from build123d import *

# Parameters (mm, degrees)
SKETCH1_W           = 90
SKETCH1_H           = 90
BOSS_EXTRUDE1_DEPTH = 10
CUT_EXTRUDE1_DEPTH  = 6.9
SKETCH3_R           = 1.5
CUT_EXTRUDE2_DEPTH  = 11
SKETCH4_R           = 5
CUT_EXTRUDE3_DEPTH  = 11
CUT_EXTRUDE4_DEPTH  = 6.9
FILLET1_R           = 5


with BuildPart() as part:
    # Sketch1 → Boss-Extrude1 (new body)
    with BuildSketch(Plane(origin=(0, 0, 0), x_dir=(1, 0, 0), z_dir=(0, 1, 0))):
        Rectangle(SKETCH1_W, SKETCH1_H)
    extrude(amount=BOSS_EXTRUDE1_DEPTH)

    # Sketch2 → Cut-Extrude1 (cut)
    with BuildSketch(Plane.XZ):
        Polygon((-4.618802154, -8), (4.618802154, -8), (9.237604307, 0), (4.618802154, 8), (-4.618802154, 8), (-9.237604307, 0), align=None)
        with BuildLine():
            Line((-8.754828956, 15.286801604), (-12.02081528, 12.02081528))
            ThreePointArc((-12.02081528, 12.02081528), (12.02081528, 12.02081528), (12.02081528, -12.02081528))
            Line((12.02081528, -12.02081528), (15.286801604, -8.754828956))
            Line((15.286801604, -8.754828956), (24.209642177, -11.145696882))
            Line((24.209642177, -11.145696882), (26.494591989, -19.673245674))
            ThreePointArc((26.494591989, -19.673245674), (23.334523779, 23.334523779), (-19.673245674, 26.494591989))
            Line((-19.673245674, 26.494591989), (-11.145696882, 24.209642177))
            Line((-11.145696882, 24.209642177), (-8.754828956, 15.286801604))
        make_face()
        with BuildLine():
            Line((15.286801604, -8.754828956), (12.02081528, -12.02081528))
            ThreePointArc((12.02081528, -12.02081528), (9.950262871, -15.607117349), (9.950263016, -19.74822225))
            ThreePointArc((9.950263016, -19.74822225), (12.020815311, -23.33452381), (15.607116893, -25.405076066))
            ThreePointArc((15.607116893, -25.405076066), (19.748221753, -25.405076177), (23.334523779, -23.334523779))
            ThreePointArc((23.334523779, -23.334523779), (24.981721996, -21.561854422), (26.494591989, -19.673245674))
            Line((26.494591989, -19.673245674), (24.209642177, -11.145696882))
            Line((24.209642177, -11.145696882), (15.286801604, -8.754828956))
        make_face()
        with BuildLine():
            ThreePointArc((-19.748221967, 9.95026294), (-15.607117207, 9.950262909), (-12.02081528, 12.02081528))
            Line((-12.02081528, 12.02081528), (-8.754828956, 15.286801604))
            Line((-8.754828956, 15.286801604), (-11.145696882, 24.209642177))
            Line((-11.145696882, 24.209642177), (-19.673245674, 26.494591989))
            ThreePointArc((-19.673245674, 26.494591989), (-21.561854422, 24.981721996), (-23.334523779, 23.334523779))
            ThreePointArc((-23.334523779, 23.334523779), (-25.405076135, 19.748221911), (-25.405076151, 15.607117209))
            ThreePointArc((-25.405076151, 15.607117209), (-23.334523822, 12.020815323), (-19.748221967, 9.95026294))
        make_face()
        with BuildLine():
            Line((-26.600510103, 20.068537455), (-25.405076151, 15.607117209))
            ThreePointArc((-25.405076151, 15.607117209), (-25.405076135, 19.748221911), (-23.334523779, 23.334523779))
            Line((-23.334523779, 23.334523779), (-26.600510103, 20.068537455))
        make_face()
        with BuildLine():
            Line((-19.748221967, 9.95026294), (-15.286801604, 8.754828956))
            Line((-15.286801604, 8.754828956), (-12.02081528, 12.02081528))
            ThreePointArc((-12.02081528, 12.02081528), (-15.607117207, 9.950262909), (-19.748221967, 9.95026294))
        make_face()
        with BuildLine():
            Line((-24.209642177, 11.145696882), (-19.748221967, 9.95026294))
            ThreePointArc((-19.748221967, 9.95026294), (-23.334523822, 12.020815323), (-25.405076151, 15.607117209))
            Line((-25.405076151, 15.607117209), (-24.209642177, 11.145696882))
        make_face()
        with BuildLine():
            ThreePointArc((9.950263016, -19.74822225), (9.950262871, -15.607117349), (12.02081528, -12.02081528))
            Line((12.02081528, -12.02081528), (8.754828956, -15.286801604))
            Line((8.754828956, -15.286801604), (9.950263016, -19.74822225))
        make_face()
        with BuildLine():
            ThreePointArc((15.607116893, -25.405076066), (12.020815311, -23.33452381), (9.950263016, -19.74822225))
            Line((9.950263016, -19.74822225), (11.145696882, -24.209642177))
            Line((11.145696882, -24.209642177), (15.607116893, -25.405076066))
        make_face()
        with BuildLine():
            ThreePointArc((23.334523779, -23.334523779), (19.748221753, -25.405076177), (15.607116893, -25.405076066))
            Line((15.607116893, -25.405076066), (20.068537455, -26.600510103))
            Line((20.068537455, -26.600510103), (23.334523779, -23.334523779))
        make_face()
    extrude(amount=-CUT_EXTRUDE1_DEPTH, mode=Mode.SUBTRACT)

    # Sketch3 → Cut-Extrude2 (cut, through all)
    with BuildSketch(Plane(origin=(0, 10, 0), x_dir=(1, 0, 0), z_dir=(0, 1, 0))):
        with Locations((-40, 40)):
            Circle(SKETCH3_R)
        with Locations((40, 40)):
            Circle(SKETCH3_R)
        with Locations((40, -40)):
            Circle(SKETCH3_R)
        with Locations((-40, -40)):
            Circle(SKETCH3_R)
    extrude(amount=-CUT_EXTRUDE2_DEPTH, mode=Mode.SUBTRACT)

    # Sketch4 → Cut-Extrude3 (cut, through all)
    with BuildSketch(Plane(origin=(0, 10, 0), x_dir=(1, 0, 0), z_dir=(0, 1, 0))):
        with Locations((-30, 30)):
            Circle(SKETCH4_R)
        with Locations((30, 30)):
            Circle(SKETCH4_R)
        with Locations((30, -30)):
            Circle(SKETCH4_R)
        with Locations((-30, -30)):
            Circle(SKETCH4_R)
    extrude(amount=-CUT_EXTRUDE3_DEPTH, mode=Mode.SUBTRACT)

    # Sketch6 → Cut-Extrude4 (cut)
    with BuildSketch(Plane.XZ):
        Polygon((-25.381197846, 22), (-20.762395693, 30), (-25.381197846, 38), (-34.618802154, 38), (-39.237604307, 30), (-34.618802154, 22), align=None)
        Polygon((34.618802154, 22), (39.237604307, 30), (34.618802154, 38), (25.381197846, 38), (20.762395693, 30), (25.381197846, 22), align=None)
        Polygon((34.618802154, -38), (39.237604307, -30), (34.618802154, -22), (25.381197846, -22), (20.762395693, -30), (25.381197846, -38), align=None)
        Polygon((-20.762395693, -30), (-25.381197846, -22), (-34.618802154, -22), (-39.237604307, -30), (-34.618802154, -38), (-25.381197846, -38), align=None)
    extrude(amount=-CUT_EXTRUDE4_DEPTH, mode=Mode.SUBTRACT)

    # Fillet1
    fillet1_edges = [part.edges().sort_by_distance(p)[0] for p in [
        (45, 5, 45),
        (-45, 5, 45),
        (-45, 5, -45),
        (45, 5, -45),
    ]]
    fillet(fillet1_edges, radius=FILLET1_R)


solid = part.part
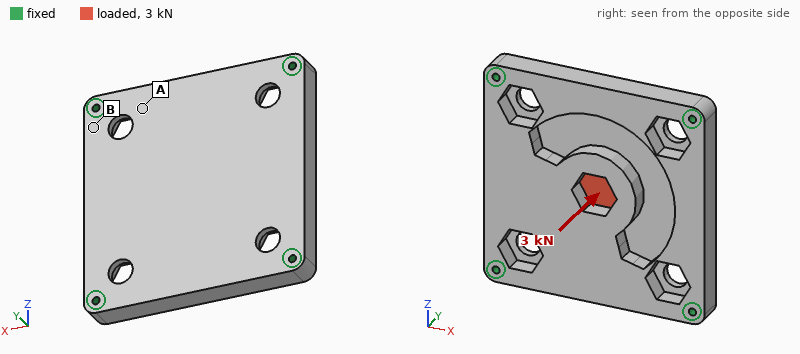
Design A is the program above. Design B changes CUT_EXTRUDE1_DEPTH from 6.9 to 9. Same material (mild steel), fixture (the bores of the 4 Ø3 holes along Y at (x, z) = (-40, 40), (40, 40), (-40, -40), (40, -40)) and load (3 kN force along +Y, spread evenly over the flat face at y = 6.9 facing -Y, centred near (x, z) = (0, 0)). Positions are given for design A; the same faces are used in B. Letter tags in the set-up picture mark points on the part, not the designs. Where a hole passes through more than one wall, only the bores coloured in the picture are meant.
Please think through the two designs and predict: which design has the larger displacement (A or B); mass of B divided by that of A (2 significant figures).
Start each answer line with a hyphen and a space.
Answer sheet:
- B
- 0.94
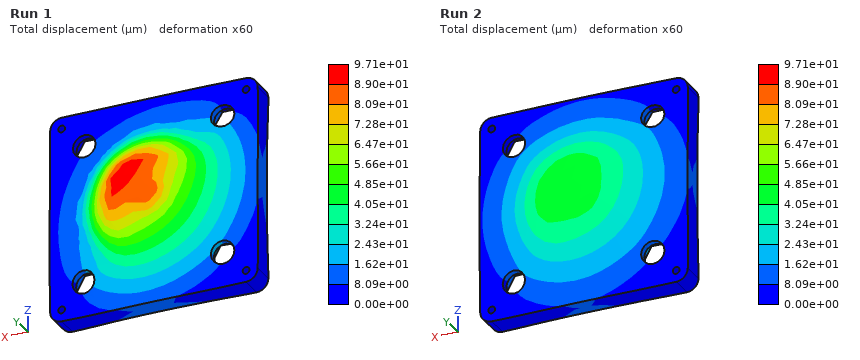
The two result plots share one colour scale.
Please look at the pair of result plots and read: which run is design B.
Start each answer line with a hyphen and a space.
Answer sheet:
- Run 1
